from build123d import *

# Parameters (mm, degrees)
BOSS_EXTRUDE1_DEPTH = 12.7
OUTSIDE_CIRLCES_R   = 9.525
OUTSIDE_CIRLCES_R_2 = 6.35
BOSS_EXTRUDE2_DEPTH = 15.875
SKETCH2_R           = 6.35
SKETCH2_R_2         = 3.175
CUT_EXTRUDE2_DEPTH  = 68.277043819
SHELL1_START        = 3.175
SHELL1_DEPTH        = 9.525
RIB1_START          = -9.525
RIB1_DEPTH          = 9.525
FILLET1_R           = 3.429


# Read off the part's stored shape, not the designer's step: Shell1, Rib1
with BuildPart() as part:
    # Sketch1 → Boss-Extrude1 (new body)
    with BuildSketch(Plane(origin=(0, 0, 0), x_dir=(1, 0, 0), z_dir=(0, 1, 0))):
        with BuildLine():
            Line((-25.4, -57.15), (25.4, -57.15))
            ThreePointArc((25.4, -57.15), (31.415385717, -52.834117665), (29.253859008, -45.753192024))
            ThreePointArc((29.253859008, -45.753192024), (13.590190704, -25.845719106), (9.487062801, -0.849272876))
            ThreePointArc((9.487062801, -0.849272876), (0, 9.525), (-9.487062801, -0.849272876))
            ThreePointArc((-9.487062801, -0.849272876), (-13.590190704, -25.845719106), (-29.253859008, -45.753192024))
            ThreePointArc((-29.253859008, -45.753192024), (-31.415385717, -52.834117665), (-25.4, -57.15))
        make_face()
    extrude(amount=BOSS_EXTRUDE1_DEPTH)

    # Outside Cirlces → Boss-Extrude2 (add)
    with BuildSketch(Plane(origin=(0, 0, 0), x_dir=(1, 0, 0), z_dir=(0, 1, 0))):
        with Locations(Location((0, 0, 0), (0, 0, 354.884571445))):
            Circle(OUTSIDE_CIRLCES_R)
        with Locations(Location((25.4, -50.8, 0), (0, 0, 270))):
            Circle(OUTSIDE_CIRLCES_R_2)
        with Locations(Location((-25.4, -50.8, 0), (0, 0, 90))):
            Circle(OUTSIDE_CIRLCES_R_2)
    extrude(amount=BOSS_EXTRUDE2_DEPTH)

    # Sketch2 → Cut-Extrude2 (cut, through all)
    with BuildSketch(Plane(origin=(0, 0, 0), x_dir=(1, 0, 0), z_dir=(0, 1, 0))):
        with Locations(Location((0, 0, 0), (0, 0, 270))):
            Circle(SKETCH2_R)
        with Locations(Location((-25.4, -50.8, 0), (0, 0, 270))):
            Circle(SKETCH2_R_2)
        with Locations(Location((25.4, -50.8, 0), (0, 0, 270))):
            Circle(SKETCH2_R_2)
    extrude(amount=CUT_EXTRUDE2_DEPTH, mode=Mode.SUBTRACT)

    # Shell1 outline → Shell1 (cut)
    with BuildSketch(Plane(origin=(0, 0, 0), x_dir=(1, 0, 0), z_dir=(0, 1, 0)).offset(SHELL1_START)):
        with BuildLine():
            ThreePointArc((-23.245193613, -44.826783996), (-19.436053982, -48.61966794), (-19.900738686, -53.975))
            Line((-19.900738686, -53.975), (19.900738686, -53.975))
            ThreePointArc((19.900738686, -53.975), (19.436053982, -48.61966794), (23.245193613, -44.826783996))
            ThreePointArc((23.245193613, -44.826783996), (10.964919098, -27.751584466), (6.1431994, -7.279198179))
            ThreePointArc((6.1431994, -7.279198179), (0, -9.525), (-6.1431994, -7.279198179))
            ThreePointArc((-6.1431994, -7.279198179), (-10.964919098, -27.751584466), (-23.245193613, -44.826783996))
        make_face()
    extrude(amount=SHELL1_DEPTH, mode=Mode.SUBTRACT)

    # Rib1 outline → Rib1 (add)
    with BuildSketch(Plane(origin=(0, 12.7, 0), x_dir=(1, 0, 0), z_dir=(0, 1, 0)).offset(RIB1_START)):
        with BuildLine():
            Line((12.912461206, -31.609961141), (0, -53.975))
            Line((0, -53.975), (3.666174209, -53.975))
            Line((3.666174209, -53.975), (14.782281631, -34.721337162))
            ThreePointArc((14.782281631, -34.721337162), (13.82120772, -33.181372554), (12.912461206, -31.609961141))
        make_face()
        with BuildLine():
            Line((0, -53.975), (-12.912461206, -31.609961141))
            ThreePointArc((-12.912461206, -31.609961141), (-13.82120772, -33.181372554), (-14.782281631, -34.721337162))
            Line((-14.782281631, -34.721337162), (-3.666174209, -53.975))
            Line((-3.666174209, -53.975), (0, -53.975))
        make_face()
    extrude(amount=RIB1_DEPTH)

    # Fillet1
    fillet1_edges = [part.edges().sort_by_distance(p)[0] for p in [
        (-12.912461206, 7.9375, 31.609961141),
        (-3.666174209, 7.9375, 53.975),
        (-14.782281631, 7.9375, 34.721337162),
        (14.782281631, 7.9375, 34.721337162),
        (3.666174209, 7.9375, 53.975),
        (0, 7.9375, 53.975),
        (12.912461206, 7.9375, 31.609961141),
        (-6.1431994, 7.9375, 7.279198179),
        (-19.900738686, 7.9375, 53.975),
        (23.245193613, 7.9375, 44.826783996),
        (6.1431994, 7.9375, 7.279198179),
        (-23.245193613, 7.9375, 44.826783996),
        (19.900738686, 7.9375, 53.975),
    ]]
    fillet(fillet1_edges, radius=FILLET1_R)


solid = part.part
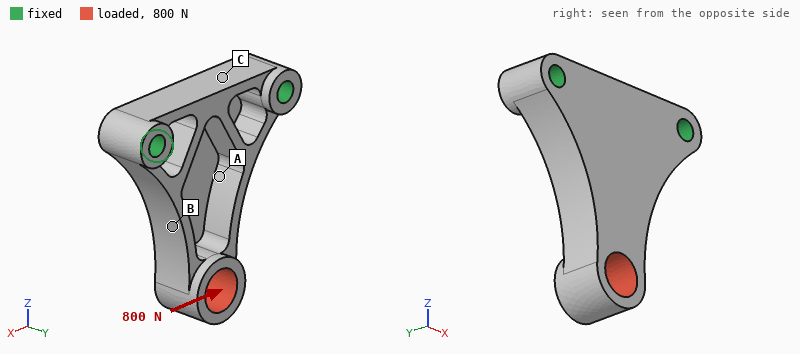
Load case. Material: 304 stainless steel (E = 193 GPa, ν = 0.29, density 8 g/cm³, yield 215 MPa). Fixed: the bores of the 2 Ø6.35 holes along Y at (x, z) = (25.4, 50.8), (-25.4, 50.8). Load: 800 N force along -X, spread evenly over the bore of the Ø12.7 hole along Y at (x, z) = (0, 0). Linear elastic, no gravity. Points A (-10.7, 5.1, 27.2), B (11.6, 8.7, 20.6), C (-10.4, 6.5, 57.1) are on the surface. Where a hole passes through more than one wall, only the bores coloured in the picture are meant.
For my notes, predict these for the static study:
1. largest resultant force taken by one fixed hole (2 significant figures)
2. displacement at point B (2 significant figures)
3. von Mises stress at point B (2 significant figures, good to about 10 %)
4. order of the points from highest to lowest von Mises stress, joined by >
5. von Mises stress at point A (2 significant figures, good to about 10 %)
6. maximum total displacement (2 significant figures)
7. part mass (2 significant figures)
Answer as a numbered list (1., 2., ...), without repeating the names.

1. 890 N
2. 5.6 µm
3. 38 MPa
4. B > A > C
5. 13 MPa
6. 25 µm
7. 130 g
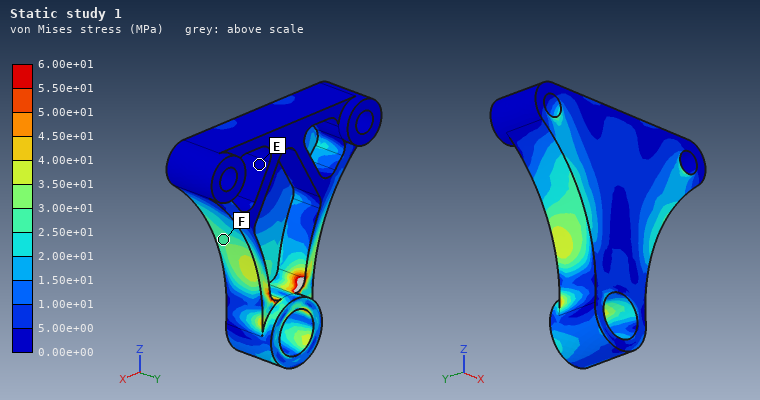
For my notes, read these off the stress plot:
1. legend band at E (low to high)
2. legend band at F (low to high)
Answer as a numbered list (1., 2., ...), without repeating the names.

1. 0.00e+00 to 5.00e+00 MPa
2. 2.50e+01 to 3.00e+01 MPa
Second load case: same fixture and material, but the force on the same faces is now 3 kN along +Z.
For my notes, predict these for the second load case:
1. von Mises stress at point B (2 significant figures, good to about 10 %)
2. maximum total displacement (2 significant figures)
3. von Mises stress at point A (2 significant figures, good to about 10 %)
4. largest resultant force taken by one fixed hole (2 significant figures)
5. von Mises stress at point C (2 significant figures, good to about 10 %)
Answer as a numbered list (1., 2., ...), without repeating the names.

1. 68 MPa
2. 53 µm
3. 33 MPa
4. 1.7 kN
5. 16 MPa
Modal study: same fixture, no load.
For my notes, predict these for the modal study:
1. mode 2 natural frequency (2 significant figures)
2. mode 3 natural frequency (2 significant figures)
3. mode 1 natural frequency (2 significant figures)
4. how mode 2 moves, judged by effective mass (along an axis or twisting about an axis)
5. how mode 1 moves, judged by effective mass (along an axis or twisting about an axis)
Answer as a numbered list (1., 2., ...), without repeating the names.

1. 6300 Hz
2. 9300 Hz
3. 2700 Hz
4. along X
5. along Y
